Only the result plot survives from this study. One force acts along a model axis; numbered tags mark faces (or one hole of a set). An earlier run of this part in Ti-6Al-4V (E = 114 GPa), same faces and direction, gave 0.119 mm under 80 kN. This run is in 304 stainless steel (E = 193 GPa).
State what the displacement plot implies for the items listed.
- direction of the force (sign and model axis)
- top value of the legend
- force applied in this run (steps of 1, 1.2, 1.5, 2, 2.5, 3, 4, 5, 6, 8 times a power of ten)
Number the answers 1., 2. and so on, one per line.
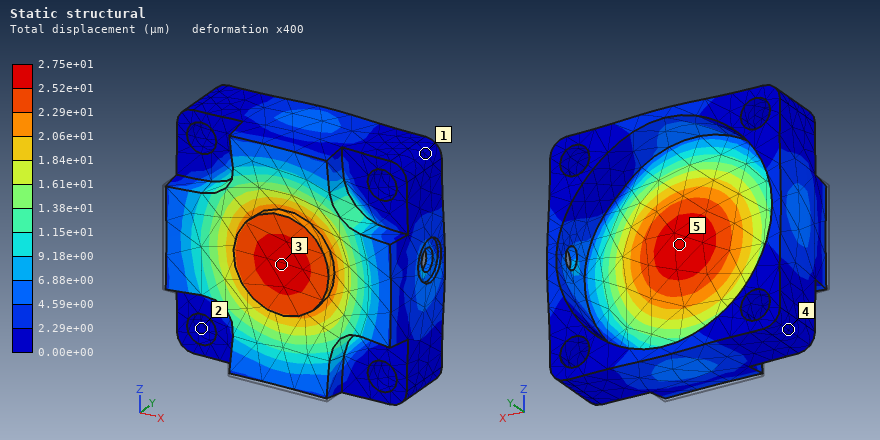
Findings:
1. +Y
2. 2.75e+01 µm
3. 30 kN
